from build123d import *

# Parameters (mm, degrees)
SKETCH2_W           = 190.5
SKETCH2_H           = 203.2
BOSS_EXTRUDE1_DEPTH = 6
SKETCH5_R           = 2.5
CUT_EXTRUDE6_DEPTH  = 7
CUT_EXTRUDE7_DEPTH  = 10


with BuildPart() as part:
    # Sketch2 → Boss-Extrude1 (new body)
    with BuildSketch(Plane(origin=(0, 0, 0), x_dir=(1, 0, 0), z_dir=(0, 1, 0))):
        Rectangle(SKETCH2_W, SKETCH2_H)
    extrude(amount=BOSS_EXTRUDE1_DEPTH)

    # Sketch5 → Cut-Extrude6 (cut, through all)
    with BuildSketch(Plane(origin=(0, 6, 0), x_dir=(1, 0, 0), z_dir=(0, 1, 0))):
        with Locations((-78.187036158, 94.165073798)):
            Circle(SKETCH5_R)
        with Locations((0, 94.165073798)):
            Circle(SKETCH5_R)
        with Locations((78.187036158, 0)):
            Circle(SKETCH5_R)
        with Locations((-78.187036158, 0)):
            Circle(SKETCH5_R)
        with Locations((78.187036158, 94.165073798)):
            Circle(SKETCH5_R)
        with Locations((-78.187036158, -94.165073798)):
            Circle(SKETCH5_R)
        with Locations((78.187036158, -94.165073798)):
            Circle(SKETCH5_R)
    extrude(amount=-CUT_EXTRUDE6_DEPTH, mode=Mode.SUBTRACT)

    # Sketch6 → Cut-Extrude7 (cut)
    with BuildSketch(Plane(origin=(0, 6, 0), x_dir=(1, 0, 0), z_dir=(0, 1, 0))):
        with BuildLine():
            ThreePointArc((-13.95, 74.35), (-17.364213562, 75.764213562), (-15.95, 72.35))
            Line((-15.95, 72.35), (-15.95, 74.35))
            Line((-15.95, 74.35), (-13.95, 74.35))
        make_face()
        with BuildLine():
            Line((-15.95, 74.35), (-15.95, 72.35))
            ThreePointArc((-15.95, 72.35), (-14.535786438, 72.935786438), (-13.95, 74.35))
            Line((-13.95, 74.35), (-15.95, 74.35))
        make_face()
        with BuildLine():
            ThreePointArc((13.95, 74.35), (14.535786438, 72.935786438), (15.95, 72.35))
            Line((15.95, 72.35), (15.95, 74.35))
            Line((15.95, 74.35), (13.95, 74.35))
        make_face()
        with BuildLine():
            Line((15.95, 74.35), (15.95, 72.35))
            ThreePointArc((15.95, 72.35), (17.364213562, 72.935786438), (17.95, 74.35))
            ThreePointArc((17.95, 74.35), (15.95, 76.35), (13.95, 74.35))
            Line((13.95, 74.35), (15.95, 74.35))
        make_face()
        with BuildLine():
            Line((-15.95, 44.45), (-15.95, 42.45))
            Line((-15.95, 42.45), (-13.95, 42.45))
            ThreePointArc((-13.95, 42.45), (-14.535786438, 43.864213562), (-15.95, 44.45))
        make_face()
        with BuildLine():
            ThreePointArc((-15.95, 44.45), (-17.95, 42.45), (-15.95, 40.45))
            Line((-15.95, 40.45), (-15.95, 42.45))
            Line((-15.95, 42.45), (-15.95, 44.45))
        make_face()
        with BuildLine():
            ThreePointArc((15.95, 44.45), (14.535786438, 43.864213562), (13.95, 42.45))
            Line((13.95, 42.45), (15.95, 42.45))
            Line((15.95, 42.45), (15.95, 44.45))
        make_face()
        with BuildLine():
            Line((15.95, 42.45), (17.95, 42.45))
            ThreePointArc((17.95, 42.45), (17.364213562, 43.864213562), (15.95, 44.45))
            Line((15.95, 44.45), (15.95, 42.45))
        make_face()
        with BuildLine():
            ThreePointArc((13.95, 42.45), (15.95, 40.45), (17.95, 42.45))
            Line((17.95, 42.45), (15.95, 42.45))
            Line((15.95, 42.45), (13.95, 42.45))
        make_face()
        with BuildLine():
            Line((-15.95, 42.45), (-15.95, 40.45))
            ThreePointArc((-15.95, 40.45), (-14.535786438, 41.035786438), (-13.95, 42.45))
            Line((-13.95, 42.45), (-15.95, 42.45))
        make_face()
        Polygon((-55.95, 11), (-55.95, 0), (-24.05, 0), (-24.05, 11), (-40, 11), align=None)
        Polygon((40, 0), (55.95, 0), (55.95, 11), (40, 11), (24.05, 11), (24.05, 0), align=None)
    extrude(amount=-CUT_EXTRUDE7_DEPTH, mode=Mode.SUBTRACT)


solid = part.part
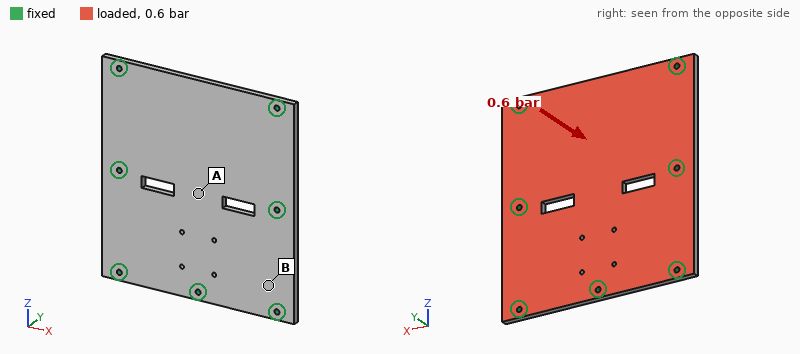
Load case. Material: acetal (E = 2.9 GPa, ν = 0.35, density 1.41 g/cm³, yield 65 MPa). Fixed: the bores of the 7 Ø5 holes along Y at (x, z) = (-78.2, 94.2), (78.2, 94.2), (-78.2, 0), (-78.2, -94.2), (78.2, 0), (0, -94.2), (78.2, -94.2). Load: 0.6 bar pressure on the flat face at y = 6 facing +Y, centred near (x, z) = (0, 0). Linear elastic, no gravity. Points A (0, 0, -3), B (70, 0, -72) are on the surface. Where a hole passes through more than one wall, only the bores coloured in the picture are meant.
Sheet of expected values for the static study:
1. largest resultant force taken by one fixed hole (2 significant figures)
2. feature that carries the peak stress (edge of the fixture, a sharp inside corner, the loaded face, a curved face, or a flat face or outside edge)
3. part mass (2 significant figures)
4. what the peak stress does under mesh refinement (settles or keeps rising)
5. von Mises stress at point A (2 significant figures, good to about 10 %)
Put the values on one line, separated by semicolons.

500 N; edge of the fixture; 320 g; keeps rising; 8.9 MPa
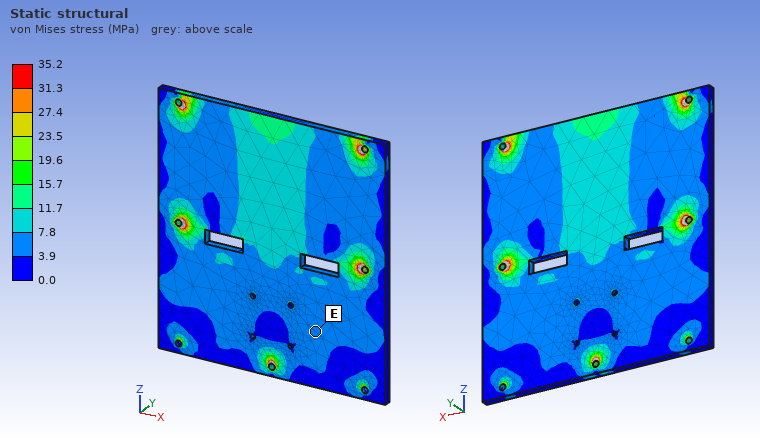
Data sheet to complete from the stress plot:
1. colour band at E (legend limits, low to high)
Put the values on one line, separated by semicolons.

3.9 to 7.8 MPa
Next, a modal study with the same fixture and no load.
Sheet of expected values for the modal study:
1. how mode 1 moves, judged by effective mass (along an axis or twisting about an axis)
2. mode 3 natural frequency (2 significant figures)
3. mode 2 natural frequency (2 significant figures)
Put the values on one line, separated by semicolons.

along Y; 720 Hz; 480 Hz
